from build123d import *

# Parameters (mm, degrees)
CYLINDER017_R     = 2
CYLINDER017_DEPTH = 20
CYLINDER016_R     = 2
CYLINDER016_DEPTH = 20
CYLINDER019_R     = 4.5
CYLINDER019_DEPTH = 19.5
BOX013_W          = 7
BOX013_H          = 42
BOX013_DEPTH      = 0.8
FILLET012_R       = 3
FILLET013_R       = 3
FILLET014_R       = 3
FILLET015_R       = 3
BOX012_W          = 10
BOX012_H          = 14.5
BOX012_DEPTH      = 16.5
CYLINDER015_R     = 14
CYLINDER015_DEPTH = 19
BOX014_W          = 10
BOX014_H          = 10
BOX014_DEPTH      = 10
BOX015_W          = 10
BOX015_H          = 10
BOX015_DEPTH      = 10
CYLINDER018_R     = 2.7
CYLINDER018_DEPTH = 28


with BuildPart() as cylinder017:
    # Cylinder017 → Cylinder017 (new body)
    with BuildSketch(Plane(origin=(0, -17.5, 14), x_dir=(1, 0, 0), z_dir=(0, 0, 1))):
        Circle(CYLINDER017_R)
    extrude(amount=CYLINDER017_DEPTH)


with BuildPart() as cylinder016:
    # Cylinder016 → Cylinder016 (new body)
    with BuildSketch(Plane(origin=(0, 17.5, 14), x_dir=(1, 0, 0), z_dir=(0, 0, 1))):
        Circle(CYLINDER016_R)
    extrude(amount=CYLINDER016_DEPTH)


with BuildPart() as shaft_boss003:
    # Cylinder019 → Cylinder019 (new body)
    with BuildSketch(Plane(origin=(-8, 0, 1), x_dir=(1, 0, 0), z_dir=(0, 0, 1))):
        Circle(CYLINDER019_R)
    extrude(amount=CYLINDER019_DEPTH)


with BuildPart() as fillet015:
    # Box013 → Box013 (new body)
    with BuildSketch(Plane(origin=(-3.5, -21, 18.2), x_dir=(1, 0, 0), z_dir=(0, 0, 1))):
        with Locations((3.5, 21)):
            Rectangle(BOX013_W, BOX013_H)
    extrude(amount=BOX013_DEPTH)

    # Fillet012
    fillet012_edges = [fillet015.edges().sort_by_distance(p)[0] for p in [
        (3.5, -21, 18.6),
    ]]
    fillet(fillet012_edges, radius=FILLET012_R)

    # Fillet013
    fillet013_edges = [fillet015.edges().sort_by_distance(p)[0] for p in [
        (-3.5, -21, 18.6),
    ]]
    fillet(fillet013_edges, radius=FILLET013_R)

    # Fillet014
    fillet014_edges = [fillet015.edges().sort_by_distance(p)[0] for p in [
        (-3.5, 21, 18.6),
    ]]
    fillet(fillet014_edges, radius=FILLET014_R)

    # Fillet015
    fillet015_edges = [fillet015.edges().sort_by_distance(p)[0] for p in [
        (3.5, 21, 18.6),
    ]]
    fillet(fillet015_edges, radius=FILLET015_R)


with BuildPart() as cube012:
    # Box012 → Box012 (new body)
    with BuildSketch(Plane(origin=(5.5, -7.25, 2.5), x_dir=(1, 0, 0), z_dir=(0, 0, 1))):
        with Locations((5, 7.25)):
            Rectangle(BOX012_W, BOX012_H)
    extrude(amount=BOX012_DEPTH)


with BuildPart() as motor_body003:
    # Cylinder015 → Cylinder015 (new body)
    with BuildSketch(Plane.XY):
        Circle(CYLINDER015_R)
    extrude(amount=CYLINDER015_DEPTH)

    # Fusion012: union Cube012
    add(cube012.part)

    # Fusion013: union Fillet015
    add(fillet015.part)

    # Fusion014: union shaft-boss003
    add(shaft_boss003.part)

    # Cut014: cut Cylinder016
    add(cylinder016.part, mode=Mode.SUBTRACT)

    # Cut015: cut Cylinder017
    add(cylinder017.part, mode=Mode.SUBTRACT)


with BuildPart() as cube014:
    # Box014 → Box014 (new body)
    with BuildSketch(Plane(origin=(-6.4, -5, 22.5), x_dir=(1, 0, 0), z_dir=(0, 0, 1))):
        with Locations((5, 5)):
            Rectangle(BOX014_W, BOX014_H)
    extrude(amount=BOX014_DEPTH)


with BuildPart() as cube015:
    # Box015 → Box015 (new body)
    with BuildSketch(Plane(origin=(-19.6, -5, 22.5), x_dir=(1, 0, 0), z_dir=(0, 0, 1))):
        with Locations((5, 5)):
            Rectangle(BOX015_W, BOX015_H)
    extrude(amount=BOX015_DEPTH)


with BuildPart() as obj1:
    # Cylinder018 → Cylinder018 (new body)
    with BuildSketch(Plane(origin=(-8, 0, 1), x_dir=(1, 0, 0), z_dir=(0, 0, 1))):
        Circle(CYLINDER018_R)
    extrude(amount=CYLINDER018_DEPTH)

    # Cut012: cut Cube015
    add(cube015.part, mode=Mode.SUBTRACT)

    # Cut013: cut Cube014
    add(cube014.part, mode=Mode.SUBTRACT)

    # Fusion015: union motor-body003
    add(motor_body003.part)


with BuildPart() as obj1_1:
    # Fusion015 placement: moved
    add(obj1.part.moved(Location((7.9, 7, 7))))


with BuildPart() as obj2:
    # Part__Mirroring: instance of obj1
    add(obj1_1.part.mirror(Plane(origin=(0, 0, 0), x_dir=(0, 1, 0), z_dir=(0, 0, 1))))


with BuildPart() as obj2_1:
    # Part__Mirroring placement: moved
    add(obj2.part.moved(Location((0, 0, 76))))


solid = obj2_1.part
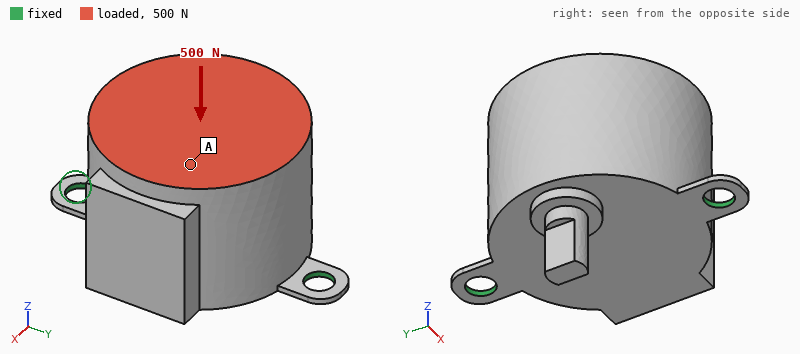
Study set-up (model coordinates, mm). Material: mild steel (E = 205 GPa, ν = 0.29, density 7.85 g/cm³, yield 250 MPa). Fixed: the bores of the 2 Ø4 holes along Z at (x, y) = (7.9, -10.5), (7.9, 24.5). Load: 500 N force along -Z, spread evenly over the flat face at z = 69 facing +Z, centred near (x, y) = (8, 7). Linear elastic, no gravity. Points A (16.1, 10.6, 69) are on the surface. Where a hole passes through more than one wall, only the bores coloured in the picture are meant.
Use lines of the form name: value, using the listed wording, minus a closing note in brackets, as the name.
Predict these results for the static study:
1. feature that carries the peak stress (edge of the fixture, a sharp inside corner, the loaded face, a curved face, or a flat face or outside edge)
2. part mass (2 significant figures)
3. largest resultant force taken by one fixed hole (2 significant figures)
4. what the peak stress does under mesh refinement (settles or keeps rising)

feature that carries the peak stress: edge of the fixture
part mass: 98 g
largest resultant force taken by one fixed hole: 290 N
what the peak stress does under mesh refinement: keeps rising
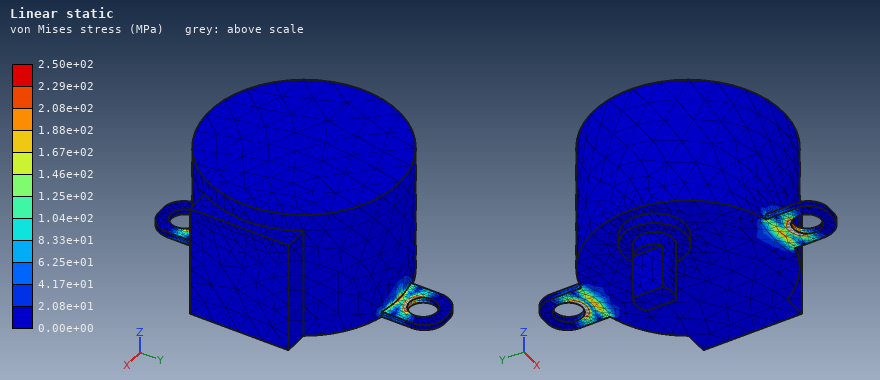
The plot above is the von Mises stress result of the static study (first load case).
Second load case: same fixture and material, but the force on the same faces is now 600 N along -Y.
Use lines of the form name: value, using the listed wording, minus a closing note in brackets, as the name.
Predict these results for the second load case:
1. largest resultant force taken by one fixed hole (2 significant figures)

largest resultant force taken by one fixed hole: 480 N
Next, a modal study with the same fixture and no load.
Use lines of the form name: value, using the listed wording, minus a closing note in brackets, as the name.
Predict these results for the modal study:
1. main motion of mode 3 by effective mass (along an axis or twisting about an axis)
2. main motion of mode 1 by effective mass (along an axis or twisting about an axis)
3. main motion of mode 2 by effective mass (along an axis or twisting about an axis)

main motion of mode 3 by effective mass: along Y
main motion of mode 1 by effective mass: along X
main motion of mode 2 by effective mass: along Z
